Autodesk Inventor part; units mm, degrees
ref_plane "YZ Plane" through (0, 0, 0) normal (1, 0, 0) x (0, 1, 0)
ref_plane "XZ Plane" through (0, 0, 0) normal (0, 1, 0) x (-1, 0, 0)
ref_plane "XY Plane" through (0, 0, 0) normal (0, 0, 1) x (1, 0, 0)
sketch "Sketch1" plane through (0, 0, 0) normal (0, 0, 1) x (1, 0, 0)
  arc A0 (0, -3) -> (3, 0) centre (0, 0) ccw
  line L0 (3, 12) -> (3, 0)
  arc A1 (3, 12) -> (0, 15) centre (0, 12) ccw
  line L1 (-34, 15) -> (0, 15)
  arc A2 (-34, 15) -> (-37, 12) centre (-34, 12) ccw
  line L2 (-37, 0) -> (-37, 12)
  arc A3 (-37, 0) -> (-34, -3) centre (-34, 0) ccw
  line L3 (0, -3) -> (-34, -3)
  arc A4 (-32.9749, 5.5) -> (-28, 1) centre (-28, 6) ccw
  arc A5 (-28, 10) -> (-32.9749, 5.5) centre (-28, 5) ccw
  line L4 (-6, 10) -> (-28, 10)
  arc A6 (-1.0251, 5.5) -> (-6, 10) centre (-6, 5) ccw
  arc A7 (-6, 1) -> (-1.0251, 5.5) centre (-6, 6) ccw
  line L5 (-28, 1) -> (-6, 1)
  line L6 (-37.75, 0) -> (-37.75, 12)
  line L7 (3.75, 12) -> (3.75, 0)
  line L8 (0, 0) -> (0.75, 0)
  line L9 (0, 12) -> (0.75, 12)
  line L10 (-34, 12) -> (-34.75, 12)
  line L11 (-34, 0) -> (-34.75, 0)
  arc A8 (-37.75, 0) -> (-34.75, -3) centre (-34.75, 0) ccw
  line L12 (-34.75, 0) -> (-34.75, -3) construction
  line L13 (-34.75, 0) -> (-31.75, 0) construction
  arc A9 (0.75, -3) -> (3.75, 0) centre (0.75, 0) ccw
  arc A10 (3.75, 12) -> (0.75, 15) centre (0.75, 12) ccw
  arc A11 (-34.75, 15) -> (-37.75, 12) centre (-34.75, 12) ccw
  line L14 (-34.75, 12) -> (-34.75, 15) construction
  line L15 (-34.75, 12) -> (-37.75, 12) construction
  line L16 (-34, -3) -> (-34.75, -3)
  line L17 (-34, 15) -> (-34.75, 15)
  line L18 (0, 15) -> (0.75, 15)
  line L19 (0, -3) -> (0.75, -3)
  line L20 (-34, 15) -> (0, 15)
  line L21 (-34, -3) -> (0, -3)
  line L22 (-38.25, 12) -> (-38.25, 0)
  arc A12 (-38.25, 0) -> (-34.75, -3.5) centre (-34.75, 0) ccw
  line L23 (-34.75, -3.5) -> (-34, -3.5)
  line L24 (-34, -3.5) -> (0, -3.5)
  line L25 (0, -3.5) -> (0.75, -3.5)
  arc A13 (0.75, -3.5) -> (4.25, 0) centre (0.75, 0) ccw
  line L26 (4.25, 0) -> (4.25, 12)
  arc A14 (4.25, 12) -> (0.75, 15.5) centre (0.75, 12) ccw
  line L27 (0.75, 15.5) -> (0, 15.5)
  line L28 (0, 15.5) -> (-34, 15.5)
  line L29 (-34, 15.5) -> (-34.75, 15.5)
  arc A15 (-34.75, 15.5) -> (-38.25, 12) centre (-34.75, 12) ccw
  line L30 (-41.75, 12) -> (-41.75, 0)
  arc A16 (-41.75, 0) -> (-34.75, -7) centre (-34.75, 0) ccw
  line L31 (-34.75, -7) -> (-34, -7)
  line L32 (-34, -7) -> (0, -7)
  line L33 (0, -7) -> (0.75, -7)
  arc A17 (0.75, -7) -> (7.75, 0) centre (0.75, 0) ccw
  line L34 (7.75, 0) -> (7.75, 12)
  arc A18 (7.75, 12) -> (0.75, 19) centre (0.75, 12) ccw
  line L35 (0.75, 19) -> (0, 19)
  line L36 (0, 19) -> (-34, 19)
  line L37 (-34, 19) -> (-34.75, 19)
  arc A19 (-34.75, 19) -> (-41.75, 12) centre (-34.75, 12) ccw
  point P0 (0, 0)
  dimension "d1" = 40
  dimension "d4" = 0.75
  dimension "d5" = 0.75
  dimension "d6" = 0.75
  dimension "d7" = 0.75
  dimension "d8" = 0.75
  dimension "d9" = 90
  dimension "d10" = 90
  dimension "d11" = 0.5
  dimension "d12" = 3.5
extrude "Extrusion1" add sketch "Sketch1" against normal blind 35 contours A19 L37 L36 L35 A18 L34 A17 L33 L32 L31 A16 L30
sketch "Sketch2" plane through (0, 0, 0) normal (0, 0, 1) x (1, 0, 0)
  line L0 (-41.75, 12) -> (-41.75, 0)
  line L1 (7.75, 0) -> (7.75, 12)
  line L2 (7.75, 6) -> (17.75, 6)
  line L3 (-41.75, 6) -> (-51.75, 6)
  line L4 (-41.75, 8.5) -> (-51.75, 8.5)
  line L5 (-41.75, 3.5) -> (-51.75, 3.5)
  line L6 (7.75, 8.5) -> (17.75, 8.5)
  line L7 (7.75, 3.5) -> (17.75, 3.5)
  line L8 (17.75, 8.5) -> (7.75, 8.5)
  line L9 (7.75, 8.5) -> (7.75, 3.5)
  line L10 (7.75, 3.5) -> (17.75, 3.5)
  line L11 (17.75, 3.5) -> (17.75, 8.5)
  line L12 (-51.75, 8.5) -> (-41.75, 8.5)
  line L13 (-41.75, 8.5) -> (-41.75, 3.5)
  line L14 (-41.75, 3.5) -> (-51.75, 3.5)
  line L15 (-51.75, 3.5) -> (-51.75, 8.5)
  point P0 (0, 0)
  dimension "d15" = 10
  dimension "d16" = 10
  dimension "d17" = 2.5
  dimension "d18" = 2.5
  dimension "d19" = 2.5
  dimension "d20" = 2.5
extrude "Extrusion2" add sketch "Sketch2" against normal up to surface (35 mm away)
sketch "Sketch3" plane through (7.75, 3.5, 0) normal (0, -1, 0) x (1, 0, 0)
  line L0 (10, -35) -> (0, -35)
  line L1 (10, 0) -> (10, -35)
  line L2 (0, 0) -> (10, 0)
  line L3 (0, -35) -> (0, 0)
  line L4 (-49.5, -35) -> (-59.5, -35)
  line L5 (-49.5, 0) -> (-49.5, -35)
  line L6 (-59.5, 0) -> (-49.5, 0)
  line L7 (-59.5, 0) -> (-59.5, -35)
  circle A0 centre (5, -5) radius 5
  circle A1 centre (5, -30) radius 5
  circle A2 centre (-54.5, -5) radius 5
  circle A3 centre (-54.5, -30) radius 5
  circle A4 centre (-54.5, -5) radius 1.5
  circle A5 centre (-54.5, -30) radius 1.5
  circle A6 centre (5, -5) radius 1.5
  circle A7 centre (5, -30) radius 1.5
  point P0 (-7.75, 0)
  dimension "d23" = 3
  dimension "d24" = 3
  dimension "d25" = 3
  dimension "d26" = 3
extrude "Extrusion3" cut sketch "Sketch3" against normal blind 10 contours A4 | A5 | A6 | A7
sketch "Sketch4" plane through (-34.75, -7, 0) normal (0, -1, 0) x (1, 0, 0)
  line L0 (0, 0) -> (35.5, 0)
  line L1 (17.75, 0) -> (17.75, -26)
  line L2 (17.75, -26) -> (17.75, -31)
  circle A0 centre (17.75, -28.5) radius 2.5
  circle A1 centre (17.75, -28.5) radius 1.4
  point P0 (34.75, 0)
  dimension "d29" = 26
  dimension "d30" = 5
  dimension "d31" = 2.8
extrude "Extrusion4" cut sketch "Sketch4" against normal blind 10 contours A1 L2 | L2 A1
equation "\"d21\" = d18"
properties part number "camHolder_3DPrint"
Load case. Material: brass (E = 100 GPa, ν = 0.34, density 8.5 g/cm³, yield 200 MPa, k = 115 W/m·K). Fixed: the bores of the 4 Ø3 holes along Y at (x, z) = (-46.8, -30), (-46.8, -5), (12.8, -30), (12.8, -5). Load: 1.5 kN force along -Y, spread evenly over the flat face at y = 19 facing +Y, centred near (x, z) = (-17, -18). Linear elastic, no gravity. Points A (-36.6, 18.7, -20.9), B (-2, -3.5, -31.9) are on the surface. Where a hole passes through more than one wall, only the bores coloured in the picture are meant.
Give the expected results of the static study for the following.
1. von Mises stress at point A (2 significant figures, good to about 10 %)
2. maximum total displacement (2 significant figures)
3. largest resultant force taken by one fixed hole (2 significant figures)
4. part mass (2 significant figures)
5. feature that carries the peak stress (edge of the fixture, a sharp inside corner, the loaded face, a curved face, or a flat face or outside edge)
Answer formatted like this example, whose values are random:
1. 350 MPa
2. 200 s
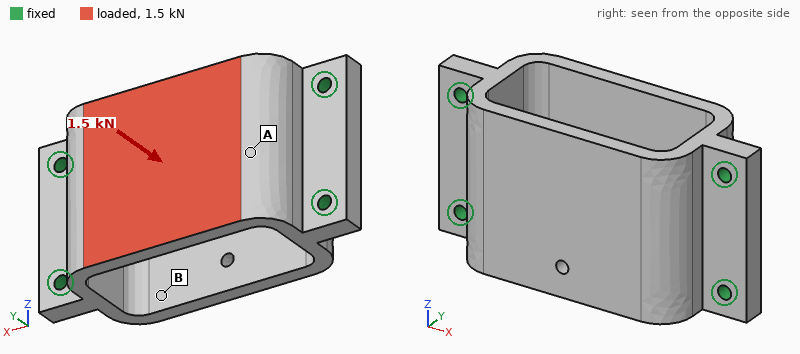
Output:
1. 30 MPa
2. 46 µm
3. 580 N
4. 160 g
5. a curved face
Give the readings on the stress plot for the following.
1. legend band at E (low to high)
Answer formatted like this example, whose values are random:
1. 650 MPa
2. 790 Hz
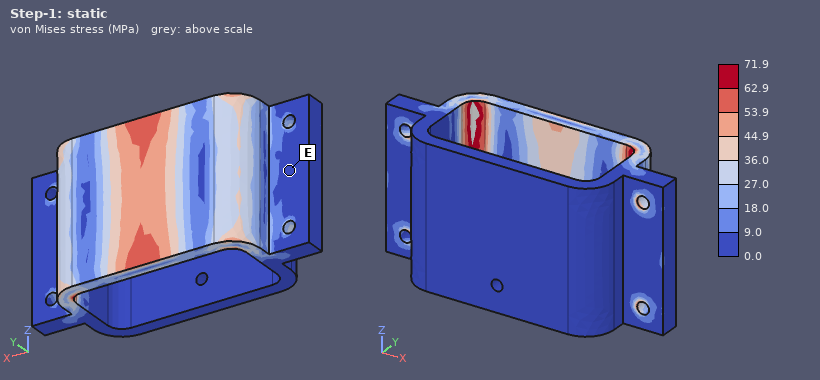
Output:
1. 0.0 to 9.0 MPa
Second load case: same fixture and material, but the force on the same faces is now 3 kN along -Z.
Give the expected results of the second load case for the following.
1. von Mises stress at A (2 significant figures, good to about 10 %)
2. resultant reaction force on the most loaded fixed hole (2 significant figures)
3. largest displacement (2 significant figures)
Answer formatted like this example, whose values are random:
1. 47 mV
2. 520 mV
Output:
1. 30 MPa
2. 1.2 kN
3. 27 µm
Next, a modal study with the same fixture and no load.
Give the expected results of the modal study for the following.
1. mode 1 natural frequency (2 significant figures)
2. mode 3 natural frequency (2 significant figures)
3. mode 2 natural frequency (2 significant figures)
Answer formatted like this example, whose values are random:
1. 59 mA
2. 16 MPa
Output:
1. 5200 Hz
2. 5600 Hz
3. 5500 Hz
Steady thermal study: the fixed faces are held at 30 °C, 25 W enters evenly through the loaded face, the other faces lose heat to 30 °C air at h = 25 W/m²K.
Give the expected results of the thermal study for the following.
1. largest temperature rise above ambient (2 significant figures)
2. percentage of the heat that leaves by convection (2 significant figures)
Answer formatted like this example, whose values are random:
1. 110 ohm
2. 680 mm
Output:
1. 23 K
2. 7.5 %
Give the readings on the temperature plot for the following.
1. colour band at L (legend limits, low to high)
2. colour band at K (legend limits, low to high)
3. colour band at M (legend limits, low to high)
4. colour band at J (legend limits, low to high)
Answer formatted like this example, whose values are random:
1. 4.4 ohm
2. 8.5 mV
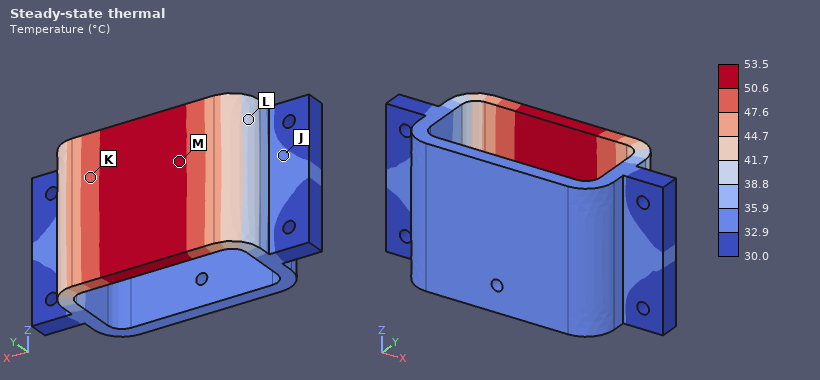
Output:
1. 38.8 to 41.7 °C
2. 47.6 to 50.6 °C
3. 50.6 to 53.5 °C
4. 32.9 to 35.9 °C
